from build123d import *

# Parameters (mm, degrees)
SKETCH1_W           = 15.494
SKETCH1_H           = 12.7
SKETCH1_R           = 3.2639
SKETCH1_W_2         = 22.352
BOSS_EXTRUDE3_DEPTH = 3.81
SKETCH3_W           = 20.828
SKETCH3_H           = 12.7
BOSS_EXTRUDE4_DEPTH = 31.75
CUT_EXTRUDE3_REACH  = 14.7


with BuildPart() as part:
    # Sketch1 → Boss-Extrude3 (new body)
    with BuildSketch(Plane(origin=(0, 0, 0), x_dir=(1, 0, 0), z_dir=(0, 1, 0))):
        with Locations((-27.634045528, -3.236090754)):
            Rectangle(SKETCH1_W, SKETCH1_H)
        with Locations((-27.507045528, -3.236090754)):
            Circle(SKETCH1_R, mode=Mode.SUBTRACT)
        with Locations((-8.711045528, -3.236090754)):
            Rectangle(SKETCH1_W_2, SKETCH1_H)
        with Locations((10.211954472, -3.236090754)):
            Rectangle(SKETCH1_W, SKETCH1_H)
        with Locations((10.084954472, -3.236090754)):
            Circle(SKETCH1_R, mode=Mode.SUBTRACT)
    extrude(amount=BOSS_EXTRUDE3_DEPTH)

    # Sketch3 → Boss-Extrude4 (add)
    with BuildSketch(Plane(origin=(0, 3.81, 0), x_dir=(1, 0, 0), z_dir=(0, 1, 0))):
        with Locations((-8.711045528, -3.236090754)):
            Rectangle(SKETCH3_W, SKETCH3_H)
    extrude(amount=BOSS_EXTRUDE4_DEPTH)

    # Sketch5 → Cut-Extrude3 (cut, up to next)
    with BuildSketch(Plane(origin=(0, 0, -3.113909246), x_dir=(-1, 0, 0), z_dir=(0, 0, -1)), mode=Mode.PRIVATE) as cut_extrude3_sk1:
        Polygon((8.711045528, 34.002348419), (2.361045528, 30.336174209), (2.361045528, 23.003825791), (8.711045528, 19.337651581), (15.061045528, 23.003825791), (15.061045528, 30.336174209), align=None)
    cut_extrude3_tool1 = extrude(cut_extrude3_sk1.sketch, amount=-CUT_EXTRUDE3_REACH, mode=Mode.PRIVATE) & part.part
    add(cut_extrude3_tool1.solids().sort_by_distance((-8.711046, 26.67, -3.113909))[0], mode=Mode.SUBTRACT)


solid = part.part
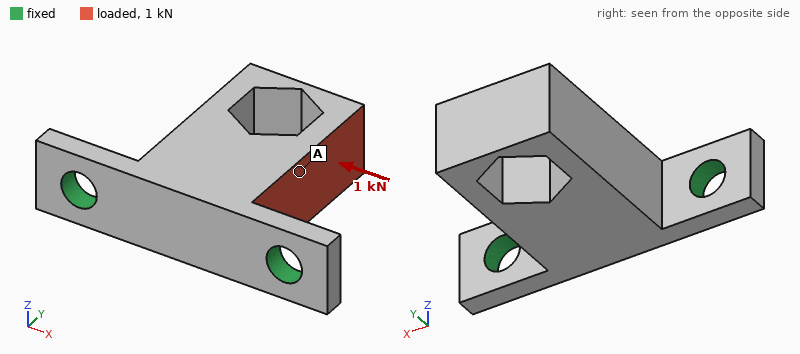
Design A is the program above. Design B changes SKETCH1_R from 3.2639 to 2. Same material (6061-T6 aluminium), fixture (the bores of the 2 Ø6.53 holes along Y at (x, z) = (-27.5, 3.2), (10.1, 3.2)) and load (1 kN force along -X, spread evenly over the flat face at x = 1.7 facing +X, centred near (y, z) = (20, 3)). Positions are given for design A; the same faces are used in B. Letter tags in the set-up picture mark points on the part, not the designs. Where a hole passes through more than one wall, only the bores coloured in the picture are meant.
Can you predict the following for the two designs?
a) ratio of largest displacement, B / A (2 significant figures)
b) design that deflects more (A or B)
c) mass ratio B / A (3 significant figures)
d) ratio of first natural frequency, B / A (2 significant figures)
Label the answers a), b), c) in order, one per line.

a) 1.2
b) B
c) 1.02
d) 0.86
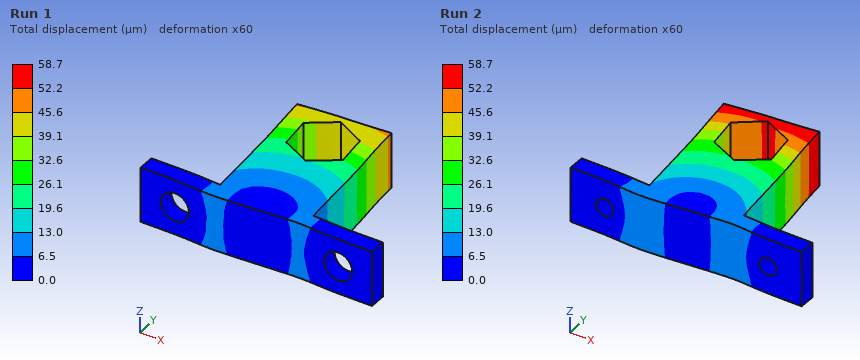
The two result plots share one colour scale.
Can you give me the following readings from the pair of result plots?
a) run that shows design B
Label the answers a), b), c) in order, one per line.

a) Run 2
